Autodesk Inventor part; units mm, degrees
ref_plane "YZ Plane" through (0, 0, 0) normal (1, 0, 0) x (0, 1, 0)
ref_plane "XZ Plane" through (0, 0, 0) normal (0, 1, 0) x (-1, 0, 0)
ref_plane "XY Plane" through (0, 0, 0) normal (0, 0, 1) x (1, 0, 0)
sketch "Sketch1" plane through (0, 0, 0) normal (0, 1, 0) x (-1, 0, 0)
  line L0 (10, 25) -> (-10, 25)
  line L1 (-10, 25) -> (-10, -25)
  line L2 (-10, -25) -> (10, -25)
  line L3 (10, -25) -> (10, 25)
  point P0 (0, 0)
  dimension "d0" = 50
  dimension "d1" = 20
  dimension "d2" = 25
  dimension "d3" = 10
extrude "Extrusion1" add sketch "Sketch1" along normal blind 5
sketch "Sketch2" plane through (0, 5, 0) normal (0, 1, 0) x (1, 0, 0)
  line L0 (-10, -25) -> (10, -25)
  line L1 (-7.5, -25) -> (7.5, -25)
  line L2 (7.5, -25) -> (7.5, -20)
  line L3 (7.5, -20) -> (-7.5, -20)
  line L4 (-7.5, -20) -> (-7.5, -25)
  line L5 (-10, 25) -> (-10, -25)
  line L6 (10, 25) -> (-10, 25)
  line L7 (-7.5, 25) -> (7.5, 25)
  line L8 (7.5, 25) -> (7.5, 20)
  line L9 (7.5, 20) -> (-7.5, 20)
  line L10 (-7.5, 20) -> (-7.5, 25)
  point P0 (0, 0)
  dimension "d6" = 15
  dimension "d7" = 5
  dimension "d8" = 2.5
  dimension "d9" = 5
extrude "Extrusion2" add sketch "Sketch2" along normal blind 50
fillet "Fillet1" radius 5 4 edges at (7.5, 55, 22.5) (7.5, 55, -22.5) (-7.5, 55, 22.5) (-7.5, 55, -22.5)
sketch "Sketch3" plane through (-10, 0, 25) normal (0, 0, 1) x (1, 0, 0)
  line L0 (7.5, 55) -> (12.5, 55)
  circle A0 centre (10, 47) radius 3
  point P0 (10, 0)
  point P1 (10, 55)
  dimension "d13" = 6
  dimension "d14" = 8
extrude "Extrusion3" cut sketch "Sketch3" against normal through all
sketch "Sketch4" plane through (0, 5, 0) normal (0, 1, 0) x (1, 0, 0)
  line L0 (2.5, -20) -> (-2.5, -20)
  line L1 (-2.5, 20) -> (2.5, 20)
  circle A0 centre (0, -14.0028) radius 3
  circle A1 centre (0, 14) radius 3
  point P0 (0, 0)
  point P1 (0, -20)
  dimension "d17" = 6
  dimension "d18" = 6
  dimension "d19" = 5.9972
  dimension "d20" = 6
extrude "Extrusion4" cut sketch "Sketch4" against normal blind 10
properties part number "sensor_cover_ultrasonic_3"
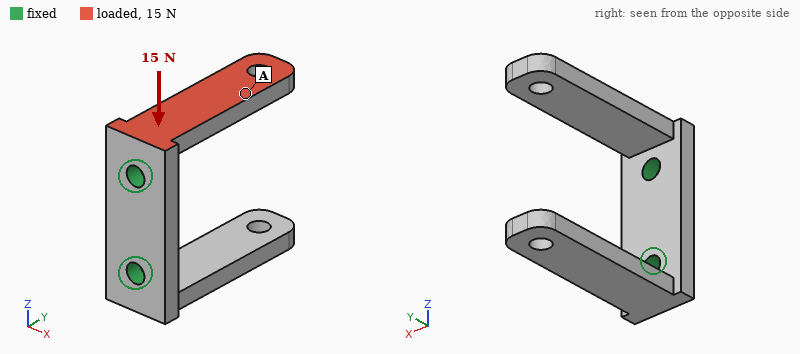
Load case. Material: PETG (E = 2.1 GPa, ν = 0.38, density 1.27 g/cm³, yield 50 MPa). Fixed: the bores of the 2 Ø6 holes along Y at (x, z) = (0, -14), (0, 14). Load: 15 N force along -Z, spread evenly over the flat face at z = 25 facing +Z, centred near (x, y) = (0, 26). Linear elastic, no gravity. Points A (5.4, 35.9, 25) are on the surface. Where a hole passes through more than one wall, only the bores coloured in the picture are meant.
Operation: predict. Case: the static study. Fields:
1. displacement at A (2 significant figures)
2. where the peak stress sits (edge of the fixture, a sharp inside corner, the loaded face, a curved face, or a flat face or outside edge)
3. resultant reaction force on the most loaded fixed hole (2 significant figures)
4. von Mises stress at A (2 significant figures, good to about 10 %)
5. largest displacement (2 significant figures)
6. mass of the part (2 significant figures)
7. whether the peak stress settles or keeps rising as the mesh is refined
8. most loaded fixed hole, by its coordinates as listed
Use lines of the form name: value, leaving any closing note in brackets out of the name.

displacement at A: 0.51 mm
where the peak stress sits: edge of the fixture
resultant reaction force on the most loaded fixed hole: 15 N
von Mises stress at A: 0.69 MPa
largest displacement: 0.92 mm
mass of the part: 15 g
whether the peak stress settles or keeps rising as the mesh is refined: keeps rising
most loaded fixed hole, by its coordinates as listed: (0, 14)
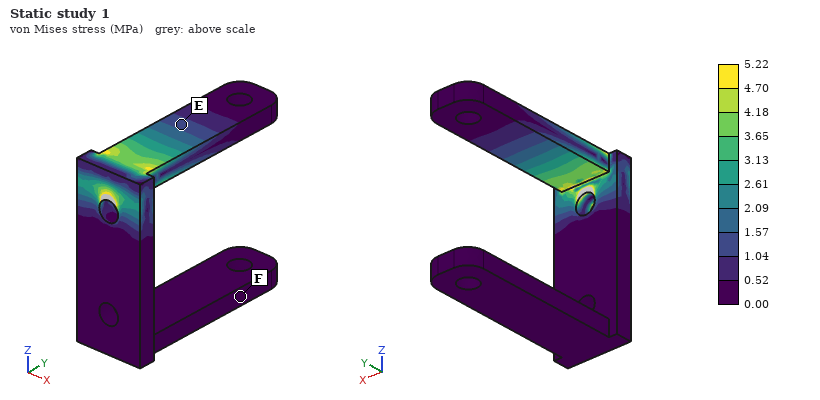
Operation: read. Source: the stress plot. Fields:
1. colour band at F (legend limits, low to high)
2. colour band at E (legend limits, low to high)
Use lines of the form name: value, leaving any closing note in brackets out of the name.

colour band at F: 0.00 to 0.52 MPa
colour band at E: 1.04 to 1.57 MPa
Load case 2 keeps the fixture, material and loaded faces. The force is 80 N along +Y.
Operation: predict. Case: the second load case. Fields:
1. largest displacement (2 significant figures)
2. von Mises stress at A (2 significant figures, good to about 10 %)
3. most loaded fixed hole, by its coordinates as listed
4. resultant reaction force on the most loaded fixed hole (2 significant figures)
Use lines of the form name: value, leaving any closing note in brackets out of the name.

largest displacement: 0.91 mm
von Mises stress at A: 1.3 MPa
most loaded fixed hole, by its coordinates as listed: (0, 14)
resultant reaction force on the most loaded fixed hole: 83 N
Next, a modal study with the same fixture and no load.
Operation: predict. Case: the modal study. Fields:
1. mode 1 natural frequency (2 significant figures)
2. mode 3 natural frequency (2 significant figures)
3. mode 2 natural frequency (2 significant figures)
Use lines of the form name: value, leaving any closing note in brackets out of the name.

mode 1 natural frequency: 360 Hz
mode 3 natural frequency: 690 Hz
mode 2 natural frequency: 360 Hz
